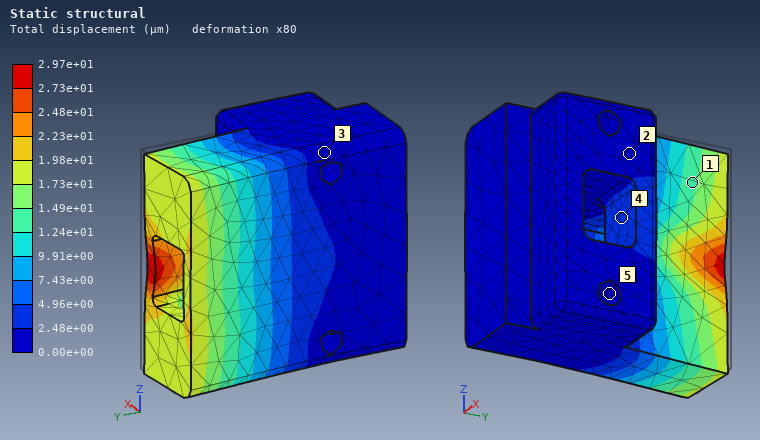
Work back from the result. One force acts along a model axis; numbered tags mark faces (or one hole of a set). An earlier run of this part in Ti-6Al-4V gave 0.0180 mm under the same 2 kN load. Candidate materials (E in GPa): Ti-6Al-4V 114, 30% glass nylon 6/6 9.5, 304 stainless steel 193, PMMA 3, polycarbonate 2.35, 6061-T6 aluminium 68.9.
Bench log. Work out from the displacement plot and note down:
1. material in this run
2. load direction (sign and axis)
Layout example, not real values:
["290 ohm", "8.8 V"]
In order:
["6061-T6 aluminium", "-X"]
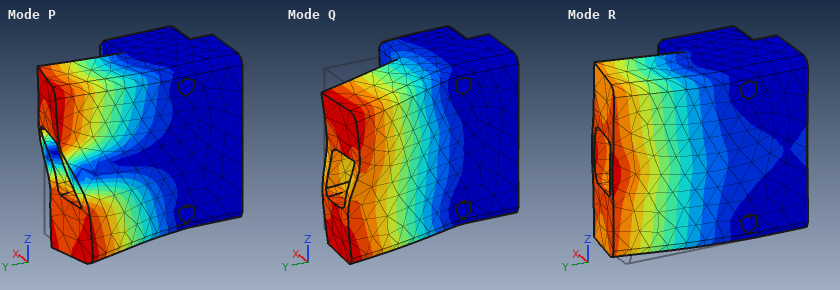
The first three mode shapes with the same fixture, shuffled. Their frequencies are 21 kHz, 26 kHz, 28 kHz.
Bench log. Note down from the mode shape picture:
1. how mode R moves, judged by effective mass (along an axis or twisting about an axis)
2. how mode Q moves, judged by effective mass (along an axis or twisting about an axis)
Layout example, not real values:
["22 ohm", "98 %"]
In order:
["along X", "along Z"]
